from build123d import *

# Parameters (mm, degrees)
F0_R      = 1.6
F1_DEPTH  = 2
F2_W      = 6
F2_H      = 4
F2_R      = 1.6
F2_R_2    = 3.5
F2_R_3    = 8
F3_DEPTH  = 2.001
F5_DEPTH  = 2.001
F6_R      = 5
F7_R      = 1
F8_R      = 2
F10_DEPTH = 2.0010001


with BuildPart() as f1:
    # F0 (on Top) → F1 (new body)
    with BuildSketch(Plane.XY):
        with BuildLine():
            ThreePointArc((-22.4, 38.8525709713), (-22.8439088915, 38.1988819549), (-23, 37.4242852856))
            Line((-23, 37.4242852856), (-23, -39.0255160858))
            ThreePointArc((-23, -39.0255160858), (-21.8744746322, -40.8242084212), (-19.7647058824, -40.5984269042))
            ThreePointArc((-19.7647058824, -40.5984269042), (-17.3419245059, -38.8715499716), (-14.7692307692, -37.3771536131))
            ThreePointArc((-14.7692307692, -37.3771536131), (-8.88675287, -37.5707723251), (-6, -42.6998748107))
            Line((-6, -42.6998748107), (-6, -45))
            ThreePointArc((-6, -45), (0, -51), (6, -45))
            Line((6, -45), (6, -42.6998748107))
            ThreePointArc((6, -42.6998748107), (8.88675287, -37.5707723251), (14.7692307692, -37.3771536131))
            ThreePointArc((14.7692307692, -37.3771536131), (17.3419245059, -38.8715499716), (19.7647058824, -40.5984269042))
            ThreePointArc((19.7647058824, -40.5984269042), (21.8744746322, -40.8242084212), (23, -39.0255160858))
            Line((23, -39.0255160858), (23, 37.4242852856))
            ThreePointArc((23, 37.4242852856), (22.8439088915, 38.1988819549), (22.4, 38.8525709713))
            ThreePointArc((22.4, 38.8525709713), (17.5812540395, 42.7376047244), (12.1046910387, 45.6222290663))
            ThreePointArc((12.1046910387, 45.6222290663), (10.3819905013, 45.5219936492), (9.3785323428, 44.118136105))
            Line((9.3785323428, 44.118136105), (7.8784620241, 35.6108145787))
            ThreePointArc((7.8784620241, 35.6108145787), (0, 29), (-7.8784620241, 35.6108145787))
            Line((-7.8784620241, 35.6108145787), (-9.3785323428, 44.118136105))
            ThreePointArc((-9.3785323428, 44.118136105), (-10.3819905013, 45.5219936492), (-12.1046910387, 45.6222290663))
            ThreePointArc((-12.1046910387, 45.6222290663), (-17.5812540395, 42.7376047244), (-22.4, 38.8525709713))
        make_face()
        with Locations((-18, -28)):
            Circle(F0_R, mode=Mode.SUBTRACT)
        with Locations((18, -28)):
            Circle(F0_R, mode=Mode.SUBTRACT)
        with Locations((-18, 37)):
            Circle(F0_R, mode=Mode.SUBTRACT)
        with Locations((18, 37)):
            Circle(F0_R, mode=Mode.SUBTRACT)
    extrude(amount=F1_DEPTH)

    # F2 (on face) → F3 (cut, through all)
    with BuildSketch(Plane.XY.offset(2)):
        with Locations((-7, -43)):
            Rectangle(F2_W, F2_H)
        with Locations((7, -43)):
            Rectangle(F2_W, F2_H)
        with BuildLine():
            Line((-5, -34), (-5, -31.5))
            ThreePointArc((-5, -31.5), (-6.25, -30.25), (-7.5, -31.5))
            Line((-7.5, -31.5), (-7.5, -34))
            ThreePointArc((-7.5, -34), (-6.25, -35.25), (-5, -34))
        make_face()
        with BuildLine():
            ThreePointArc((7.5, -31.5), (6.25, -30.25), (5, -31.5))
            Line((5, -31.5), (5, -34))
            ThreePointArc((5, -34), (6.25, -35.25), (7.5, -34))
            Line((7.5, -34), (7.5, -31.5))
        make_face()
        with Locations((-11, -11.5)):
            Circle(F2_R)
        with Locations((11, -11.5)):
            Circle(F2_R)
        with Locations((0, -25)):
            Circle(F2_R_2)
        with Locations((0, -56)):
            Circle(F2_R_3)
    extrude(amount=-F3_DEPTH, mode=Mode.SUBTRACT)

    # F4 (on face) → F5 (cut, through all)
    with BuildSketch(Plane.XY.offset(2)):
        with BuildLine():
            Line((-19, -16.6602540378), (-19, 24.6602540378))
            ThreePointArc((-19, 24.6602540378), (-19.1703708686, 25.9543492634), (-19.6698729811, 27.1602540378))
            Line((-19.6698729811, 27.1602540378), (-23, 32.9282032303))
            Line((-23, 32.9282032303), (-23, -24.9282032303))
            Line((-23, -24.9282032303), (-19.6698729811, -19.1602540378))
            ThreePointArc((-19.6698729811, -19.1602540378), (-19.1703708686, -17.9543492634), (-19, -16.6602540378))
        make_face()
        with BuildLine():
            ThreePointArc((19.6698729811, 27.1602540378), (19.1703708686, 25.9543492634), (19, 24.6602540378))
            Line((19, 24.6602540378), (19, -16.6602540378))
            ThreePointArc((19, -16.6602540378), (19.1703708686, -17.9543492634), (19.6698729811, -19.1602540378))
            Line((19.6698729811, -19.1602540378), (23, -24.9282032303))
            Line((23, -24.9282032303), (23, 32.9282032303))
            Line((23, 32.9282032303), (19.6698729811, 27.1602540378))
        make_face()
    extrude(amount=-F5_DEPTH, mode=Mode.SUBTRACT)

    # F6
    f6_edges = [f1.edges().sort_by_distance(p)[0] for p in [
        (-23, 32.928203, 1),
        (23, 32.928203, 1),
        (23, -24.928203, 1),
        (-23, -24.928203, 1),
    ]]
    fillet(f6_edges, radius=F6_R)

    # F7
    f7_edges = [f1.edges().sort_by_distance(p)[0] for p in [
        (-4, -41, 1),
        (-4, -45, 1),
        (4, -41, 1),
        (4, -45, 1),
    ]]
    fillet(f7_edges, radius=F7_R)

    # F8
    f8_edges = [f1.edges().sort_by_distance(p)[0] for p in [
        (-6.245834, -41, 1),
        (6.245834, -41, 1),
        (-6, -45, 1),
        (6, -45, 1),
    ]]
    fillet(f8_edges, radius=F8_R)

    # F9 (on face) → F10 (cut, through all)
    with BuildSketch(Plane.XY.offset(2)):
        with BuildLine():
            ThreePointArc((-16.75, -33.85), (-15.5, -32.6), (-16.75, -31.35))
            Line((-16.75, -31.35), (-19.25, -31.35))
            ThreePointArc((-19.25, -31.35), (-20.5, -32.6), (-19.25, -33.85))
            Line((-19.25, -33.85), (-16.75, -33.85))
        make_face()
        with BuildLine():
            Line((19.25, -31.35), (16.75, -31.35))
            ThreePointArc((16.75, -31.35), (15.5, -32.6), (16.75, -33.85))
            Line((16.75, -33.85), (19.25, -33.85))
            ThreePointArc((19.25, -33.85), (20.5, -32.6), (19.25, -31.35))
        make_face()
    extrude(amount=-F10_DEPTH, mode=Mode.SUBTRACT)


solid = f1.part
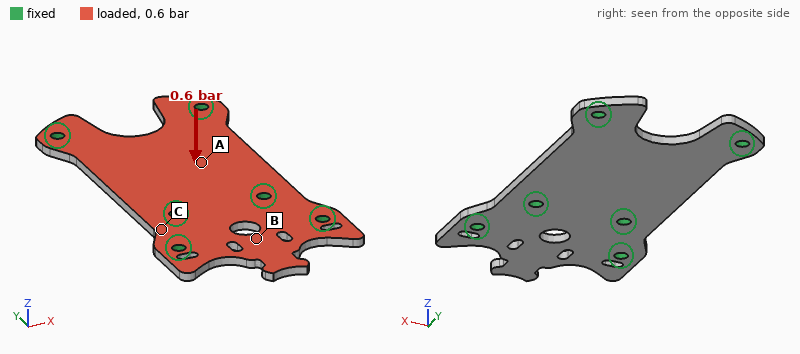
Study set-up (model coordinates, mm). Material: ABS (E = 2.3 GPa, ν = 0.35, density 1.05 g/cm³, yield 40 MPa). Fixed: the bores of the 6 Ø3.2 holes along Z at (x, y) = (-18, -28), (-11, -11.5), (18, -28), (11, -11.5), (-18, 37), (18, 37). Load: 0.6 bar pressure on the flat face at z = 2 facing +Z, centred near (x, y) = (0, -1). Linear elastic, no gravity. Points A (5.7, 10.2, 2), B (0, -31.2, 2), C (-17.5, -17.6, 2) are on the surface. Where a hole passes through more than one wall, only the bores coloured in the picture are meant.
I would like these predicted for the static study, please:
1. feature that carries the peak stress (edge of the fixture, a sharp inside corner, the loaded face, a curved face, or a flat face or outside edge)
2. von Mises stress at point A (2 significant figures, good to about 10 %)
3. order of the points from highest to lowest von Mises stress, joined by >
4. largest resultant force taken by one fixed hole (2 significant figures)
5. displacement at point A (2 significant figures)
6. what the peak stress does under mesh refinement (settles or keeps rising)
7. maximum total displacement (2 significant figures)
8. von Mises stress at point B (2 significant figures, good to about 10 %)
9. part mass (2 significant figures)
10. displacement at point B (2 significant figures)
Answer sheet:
edge of the fixture
7.5 MPa
A > B > C
39 N
0.60 mm
keeps rising
1.0 mm
5.5 MPa
6.5 g
0.25 mm
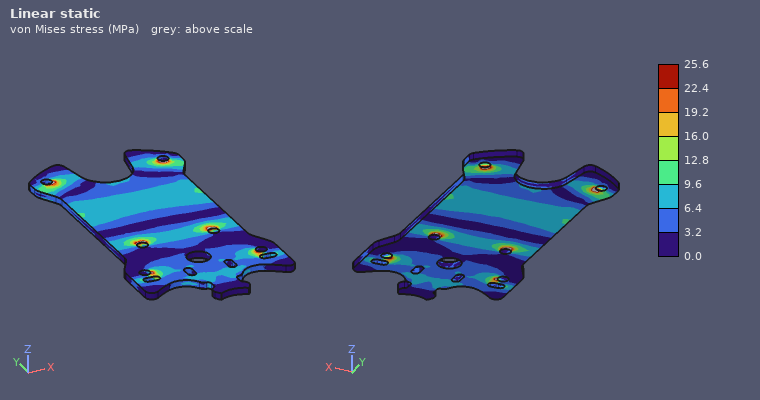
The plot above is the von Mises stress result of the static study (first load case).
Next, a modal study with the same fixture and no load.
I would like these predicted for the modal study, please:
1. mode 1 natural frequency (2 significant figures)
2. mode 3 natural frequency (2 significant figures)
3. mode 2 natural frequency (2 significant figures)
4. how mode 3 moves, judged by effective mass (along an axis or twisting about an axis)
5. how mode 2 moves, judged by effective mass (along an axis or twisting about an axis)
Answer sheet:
1200 Hz
1700 Hz
1200 Hz
twisting about Y
along Z
